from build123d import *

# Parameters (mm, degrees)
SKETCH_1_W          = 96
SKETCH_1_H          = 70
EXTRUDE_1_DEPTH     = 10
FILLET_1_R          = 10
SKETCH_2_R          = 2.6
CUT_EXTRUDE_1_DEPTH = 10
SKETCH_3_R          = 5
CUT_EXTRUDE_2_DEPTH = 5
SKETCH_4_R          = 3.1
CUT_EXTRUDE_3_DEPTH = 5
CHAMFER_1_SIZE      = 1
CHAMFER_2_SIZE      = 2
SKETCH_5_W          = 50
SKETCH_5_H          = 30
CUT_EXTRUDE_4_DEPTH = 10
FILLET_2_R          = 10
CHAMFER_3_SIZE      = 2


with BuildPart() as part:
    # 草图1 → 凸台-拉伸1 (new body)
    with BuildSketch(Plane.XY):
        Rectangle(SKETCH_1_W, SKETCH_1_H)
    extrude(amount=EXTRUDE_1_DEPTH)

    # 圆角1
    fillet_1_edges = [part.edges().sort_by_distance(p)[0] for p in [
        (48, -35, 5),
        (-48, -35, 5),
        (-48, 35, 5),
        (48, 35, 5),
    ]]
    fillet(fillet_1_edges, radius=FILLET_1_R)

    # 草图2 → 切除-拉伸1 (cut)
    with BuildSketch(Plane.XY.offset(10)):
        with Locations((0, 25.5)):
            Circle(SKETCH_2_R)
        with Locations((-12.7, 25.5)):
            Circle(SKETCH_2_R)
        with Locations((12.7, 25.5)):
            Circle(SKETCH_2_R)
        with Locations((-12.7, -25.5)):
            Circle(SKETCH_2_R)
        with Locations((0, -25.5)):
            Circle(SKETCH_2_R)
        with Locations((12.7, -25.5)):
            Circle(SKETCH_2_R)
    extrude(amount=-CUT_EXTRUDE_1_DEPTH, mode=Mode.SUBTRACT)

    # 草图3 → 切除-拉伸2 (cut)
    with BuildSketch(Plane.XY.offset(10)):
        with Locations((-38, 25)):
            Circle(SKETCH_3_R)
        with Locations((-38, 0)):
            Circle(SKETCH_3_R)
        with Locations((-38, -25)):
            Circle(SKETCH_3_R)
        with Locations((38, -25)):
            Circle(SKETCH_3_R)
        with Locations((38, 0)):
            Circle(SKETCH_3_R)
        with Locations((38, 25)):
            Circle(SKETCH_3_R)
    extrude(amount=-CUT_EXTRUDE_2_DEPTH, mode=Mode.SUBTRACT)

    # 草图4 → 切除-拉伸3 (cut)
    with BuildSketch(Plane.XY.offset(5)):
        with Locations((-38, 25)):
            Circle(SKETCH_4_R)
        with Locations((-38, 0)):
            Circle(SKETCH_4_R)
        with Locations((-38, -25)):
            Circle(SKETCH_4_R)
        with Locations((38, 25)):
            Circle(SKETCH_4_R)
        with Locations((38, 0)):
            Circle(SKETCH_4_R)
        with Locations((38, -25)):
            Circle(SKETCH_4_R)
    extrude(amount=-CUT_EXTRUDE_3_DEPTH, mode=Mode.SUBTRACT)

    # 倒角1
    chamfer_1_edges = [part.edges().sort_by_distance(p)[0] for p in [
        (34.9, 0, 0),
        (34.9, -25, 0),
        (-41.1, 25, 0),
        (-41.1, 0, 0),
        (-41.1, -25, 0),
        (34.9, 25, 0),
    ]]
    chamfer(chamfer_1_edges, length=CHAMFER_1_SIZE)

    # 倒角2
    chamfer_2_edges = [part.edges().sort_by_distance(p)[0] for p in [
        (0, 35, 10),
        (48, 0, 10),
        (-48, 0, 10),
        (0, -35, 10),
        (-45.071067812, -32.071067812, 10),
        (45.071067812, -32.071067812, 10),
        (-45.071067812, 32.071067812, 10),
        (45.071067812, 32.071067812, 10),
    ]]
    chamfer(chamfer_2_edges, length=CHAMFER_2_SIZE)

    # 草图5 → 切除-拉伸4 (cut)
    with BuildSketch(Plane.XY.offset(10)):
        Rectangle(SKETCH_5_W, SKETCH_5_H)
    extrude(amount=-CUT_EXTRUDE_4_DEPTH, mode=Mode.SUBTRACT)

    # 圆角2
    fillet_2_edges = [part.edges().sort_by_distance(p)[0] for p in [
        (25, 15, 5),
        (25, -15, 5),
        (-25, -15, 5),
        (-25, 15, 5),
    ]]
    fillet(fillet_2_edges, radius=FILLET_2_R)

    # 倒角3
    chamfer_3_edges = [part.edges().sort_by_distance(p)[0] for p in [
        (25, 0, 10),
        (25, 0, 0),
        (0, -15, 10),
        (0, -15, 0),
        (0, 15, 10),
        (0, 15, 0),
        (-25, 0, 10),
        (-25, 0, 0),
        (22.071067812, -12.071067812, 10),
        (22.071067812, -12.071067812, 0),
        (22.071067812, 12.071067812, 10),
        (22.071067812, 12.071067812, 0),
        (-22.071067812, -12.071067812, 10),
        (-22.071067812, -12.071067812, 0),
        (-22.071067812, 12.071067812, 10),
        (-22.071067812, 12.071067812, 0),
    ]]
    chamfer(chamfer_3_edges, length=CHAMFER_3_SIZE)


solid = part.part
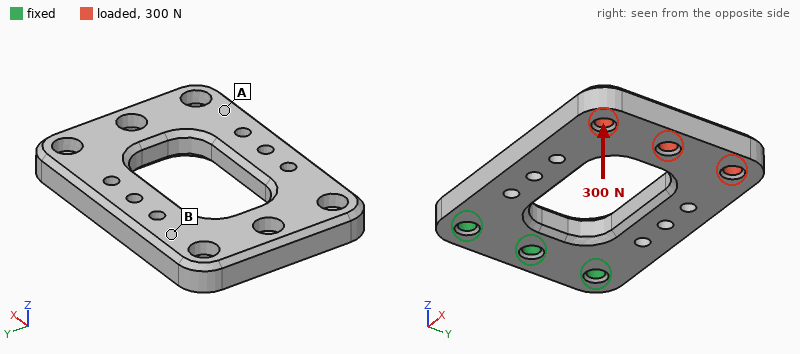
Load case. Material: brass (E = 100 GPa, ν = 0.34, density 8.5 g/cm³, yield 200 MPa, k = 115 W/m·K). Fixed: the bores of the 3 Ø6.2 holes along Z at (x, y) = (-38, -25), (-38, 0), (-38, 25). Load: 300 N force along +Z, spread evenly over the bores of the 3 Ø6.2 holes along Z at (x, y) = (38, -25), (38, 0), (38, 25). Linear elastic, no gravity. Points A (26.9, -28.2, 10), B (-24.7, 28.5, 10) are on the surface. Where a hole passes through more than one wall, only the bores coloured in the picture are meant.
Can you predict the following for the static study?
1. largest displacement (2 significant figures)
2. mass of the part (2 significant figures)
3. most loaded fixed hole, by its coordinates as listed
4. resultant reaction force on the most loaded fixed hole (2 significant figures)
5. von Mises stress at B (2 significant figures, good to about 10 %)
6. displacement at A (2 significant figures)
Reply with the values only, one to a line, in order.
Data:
0.22 mm
390 g
(-38, 0)
180 N
22 MPa
0.15 mm
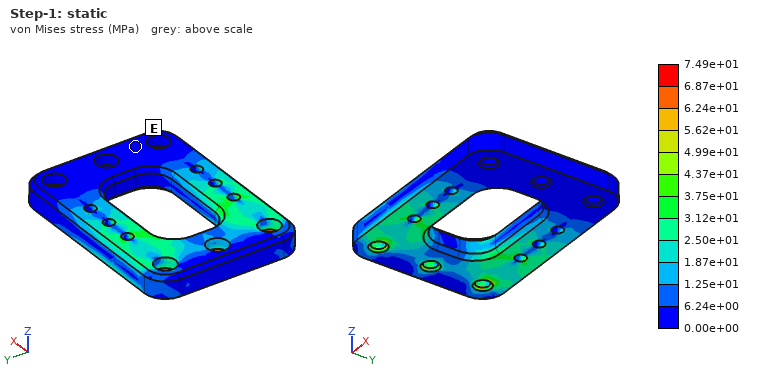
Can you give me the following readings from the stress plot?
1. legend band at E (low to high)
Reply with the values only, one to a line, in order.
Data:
0.00e+00 to 6.24e+00 MPa
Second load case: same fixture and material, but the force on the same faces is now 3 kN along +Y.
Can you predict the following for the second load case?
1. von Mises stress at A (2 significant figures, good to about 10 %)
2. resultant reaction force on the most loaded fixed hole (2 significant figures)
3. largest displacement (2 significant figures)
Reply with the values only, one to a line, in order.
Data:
14 MPa
4.2 kN
0.12 mm
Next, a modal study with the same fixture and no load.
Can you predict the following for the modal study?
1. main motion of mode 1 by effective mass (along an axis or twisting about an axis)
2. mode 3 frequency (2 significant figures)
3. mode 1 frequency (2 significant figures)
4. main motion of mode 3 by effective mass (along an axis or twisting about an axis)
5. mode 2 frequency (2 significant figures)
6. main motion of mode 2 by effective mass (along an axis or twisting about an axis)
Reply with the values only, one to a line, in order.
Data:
along Z
2200 Hz
550 Hz
along Y
1500 Hz
twisting about X
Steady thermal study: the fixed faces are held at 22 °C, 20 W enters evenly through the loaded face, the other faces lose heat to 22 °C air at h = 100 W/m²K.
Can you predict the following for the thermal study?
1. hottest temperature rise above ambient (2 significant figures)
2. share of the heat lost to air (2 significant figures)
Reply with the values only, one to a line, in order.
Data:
19 K
63 %
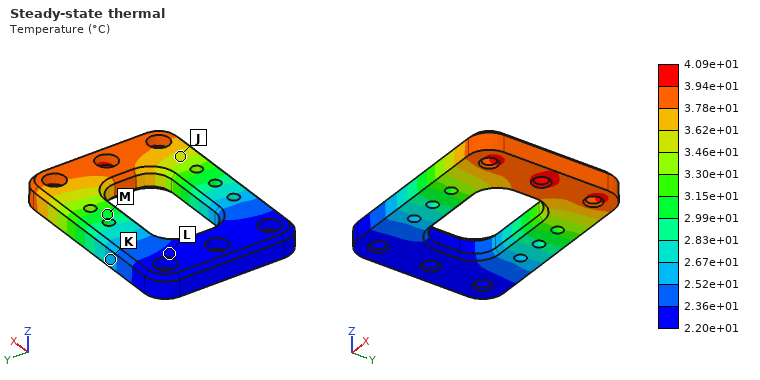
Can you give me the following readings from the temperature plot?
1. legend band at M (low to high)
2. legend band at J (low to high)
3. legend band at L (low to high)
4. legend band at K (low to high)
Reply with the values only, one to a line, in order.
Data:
2.99e+01 to 3.15e+01 °C
3.46e+01 to 3.62e+01 °C
2.20e+01 to 2.36e+01 °C
2.52e+01 to 2.67e+01 °C
